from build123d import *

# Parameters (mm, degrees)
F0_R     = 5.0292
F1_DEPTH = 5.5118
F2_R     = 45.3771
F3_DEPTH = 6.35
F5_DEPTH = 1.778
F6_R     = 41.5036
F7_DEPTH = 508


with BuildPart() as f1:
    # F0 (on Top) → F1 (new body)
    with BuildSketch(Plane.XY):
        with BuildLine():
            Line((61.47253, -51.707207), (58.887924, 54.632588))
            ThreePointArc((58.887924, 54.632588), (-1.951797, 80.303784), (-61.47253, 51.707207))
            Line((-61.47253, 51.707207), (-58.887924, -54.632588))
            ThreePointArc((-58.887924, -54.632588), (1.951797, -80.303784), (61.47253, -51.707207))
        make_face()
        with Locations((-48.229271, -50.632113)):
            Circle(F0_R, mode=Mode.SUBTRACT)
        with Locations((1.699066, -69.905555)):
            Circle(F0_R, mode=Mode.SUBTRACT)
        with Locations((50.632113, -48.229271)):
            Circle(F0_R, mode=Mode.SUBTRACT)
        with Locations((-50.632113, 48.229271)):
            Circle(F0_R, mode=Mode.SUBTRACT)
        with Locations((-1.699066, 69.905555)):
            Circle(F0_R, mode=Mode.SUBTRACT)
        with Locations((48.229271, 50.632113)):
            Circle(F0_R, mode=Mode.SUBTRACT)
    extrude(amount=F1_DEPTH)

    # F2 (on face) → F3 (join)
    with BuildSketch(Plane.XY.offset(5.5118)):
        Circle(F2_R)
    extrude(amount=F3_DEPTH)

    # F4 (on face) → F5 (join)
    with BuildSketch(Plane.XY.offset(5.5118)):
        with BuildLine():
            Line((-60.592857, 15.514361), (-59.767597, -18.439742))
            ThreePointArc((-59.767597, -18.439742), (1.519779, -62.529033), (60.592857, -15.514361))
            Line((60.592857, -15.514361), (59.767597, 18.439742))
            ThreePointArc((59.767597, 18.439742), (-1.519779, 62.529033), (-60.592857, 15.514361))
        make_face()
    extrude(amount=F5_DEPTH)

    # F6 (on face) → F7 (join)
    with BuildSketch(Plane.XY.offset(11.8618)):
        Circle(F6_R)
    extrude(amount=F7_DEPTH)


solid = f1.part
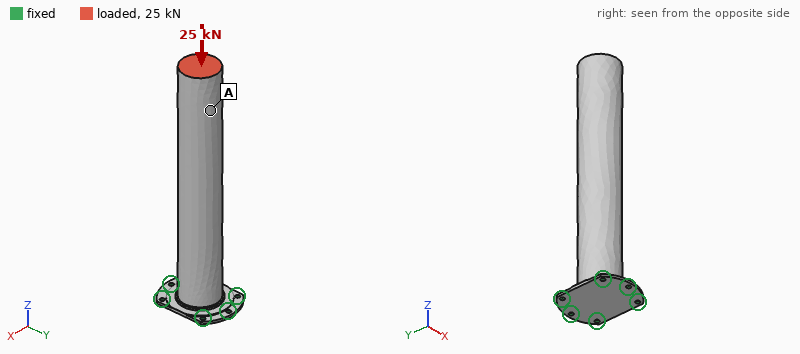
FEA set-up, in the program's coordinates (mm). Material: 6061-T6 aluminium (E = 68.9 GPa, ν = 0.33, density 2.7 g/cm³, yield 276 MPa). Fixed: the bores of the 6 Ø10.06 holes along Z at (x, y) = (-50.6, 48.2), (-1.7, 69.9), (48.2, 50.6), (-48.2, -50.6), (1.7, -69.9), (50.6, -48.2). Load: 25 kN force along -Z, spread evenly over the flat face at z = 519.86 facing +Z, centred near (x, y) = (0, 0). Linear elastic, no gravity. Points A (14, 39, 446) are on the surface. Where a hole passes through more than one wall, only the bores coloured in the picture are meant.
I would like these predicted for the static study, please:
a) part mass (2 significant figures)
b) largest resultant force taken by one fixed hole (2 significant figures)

7.8 kg
6.0 kN
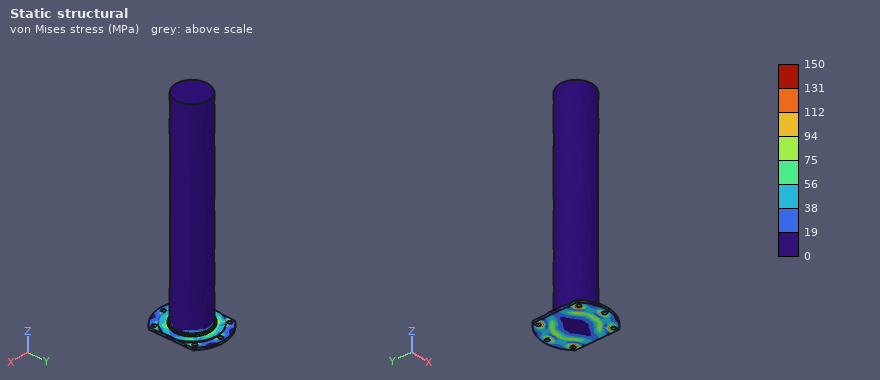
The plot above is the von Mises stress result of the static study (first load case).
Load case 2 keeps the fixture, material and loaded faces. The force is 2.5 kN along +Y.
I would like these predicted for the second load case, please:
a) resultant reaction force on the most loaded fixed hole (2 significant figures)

5.7 kN
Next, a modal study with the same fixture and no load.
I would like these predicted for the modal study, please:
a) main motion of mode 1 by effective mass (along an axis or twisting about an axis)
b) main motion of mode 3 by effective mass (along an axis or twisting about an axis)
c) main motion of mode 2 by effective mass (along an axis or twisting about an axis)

along X
along Z
along Y
